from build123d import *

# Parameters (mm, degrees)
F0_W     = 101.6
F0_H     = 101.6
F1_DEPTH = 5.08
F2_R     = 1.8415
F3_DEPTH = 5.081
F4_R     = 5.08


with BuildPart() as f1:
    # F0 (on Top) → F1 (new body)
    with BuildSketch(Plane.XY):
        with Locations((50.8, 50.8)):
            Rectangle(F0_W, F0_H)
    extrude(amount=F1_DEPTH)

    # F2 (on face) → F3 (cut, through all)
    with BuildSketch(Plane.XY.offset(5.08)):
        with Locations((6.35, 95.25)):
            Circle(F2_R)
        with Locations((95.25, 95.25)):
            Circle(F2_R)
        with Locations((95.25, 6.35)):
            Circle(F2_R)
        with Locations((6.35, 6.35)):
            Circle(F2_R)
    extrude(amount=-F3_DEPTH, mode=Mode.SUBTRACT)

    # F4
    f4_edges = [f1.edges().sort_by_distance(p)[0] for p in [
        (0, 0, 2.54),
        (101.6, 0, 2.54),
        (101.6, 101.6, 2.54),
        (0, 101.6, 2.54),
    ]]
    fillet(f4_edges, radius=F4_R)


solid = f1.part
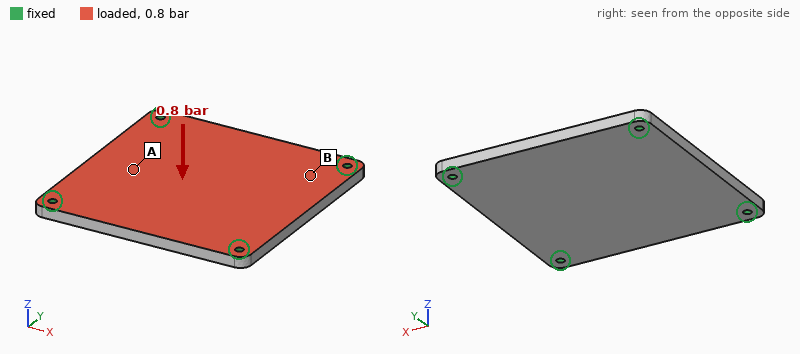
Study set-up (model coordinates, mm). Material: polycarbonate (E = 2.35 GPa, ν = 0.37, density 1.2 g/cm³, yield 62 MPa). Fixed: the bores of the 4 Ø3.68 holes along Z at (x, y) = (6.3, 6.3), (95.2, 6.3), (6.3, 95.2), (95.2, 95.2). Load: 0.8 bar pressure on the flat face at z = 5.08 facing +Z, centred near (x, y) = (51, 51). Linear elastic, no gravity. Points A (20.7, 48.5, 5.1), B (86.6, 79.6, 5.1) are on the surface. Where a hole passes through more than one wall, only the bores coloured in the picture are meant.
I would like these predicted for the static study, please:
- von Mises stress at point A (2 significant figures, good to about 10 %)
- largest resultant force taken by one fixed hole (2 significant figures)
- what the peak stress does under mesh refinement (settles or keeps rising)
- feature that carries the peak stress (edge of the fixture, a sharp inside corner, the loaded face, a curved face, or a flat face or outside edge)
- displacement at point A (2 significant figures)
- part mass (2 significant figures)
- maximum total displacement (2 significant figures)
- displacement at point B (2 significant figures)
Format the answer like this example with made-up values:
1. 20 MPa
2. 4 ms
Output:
1. 8.0 MPa
2. 210 N
3. keeps rising
4. edge of the fixture
5. 1.1 mm
6. 63 g
7. 1.5 mm
8. 0.55 mm
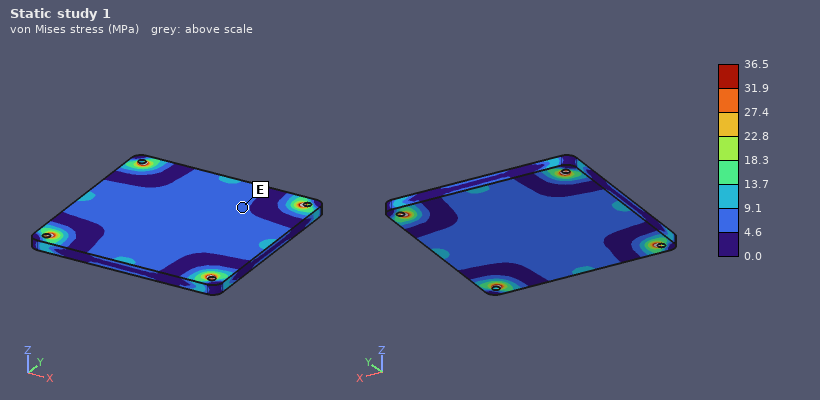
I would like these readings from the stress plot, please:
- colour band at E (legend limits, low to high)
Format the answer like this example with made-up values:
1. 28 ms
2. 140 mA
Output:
1. 4.6 to 9.1 MPa
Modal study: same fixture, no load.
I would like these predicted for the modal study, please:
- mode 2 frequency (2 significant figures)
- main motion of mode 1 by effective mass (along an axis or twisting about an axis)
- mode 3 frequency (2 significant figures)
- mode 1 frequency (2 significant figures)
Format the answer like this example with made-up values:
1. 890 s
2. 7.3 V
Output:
1. 970 Hz
2. along Z
3. 970 Hz
4. 560 Hz
